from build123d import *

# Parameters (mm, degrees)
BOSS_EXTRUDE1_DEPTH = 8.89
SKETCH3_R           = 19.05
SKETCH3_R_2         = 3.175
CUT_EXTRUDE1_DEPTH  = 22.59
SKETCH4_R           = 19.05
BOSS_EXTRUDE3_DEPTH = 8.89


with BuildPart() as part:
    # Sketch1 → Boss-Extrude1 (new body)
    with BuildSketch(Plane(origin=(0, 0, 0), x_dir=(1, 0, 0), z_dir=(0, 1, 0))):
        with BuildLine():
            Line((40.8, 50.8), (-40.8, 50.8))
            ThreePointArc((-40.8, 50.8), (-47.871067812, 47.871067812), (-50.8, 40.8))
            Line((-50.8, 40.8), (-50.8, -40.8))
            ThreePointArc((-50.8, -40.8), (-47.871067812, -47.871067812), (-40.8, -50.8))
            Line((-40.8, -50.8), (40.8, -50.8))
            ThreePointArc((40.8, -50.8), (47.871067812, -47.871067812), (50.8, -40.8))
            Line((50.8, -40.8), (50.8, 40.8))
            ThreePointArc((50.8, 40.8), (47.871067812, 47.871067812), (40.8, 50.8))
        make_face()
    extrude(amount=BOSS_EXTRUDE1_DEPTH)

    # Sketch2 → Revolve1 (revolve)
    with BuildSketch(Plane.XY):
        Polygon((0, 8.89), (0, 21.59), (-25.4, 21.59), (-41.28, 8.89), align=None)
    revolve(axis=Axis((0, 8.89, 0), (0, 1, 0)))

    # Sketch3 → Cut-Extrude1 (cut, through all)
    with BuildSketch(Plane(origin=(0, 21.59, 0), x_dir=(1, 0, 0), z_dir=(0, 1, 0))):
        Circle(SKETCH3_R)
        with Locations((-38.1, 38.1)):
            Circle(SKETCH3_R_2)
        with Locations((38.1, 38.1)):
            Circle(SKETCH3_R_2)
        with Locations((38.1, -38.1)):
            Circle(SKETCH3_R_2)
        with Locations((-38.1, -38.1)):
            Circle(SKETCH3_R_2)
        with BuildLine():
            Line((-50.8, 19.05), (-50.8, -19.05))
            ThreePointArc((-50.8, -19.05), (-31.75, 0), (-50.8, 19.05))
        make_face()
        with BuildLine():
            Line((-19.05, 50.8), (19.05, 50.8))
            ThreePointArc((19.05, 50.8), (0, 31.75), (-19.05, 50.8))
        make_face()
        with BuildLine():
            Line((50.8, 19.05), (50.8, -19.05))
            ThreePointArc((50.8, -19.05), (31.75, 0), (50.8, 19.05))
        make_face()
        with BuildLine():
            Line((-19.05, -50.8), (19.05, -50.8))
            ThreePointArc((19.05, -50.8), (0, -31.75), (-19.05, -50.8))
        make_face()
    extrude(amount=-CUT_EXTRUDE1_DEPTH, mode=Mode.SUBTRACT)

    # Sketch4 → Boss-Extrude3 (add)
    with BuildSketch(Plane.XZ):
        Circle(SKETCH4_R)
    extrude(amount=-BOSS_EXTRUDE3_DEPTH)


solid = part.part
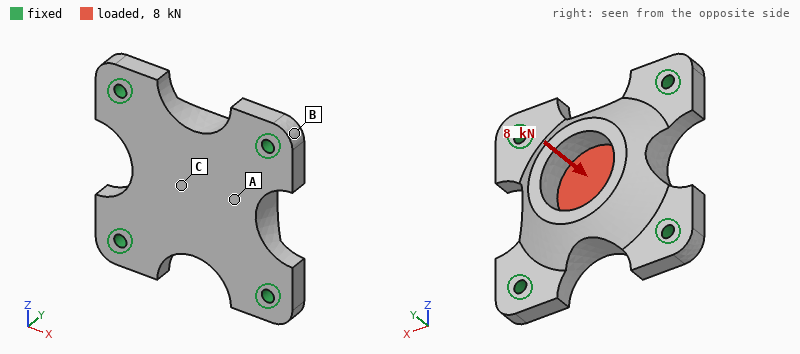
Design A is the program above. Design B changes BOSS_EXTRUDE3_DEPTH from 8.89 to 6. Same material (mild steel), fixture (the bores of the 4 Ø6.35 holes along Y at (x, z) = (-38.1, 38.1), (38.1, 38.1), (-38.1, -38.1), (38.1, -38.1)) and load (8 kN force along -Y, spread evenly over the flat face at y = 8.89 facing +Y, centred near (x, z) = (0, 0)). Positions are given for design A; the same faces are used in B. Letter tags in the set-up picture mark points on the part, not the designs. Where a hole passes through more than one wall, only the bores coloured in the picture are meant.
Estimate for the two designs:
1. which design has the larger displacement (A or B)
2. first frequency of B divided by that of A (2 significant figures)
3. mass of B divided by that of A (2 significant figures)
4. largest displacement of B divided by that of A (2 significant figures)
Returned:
B
1.0
0.97
1.3
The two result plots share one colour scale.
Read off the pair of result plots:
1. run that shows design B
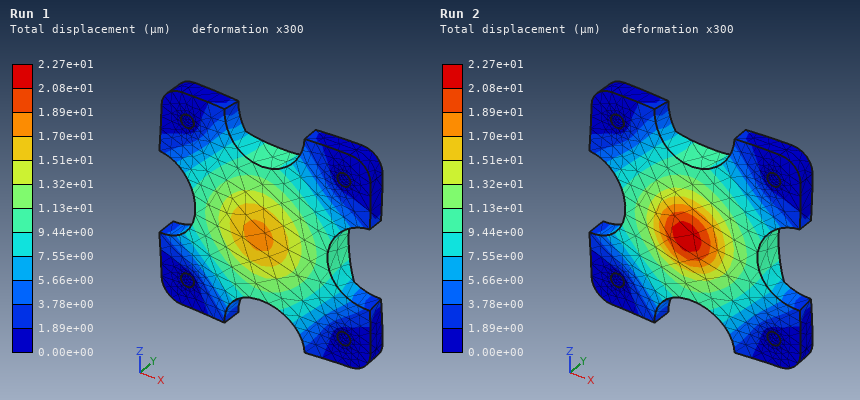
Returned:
Run 2
